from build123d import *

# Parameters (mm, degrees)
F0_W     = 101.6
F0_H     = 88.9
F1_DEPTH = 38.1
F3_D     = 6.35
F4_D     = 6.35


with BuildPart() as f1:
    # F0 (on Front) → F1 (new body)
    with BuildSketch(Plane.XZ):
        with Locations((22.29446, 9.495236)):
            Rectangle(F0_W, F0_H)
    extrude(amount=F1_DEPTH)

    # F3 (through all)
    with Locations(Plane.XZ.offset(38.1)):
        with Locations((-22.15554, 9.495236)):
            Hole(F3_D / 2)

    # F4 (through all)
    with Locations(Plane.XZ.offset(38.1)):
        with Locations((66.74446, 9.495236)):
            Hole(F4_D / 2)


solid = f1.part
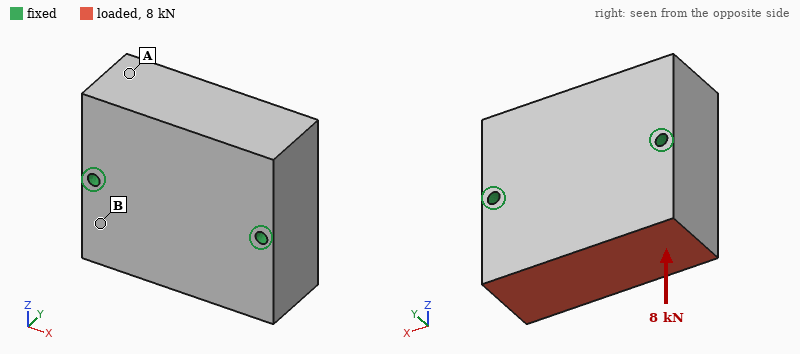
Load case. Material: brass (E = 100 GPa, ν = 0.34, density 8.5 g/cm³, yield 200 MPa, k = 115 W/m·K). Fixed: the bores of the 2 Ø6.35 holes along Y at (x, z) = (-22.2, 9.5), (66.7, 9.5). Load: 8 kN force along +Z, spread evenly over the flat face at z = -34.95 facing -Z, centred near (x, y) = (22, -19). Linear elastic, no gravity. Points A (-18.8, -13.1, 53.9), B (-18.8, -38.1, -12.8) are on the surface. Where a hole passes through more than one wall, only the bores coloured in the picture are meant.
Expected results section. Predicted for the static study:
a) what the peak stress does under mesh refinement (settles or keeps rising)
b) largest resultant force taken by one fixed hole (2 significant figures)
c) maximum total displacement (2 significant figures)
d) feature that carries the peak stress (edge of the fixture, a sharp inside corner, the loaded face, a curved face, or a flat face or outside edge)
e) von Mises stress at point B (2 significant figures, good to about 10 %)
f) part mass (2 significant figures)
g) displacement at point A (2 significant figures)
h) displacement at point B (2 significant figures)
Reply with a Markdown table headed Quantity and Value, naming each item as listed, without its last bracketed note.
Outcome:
| Quantity | Value |
|---|---|
| what the peak stress does under mesh refinement | keeps rising |
| largest resultant force taken by one fixed hole | 4.0 kN |
| maximum total displacement | 1.8 µm |
| feature that carries the peak stress | edge of the fixture |
| von Mises stress at point B | 2.8 MPa |
| part mass | 2.9 kg |
| displacement at point A | 0.61 µm |
| displacement at point B | 0.85 µm |
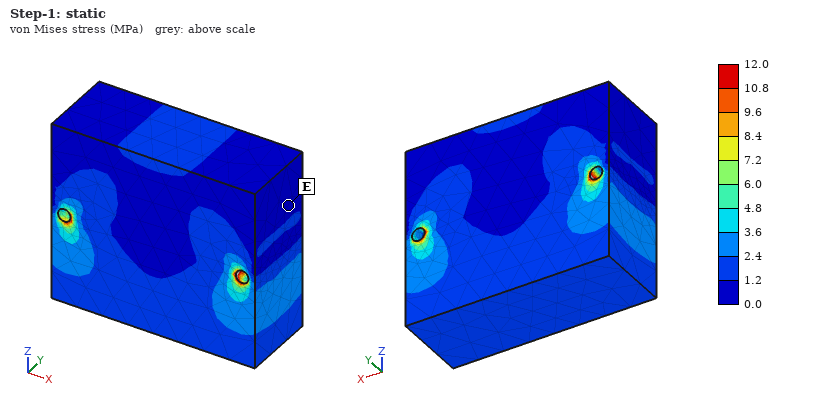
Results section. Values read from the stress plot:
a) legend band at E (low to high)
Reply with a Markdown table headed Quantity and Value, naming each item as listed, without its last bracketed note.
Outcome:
| Quantity | Value |
|---|---|
| legend band at E | 0.0 to 1.2 MPa |
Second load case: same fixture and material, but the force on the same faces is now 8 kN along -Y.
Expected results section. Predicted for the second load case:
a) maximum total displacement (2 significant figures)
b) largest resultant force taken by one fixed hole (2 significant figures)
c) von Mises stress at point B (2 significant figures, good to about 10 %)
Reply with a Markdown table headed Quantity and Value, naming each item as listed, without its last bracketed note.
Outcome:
| Quantity | Value |
|---|---|
| maximum total displacement | 18 µm |
| largest resultant force taken by one fixed hole | 4.0 kN |
| von Mises stress at point B | 10 MPa |
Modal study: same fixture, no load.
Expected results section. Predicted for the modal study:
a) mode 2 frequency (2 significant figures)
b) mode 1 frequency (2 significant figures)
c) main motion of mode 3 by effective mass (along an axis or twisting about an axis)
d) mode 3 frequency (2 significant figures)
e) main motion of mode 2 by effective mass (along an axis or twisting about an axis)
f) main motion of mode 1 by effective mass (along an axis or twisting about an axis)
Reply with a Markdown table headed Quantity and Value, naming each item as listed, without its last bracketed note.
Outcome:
| Quantity | Value |
|---|---|
| mode 2 frequency | 5300 Hz |
| mode 1 frequency | 4300 Hz |
| main motion of mode 3 by effective mass | along X |
| mode 3 frequency | 7900 Hz |
| main motion of mode 2 by effective mass | along Y |
| main motion of mode 1 by effective mass | twisting about X |
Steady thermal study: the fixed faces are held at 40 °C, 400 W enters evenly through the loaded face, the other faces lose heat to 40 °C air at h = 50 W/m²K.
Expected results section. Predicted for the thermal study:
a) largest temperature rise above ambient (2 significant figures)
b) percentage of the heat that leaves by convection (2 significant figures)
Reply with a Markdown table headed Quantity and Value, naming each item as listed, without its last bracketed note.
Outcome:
| Quantity | Value |
|---|---|
| largest temperature rise above ambient | 53 K |
| percentage of the heat that leaves by convection | 7.0 % |
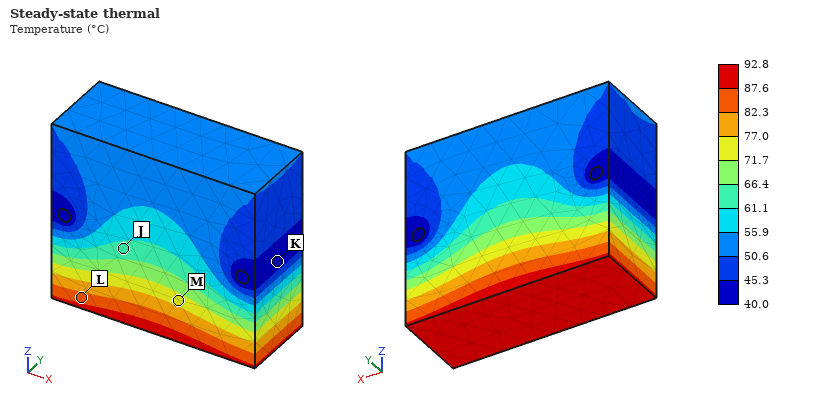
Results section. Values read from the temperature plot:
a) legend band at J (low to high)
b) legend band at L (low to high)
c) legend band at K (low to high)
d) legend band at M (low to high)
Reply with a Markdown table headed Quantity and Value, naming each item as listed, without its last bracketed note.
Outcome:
| Quantity | Value |
|---|---|
| legend band at J | 61.1 to 66.4 °C |
| legend band at L | 82.3 to 87.6 °C |
| legend band at K | 40.0 to 45.3 °C |
| legend band at M | 71.7 to 77.0 °C |
